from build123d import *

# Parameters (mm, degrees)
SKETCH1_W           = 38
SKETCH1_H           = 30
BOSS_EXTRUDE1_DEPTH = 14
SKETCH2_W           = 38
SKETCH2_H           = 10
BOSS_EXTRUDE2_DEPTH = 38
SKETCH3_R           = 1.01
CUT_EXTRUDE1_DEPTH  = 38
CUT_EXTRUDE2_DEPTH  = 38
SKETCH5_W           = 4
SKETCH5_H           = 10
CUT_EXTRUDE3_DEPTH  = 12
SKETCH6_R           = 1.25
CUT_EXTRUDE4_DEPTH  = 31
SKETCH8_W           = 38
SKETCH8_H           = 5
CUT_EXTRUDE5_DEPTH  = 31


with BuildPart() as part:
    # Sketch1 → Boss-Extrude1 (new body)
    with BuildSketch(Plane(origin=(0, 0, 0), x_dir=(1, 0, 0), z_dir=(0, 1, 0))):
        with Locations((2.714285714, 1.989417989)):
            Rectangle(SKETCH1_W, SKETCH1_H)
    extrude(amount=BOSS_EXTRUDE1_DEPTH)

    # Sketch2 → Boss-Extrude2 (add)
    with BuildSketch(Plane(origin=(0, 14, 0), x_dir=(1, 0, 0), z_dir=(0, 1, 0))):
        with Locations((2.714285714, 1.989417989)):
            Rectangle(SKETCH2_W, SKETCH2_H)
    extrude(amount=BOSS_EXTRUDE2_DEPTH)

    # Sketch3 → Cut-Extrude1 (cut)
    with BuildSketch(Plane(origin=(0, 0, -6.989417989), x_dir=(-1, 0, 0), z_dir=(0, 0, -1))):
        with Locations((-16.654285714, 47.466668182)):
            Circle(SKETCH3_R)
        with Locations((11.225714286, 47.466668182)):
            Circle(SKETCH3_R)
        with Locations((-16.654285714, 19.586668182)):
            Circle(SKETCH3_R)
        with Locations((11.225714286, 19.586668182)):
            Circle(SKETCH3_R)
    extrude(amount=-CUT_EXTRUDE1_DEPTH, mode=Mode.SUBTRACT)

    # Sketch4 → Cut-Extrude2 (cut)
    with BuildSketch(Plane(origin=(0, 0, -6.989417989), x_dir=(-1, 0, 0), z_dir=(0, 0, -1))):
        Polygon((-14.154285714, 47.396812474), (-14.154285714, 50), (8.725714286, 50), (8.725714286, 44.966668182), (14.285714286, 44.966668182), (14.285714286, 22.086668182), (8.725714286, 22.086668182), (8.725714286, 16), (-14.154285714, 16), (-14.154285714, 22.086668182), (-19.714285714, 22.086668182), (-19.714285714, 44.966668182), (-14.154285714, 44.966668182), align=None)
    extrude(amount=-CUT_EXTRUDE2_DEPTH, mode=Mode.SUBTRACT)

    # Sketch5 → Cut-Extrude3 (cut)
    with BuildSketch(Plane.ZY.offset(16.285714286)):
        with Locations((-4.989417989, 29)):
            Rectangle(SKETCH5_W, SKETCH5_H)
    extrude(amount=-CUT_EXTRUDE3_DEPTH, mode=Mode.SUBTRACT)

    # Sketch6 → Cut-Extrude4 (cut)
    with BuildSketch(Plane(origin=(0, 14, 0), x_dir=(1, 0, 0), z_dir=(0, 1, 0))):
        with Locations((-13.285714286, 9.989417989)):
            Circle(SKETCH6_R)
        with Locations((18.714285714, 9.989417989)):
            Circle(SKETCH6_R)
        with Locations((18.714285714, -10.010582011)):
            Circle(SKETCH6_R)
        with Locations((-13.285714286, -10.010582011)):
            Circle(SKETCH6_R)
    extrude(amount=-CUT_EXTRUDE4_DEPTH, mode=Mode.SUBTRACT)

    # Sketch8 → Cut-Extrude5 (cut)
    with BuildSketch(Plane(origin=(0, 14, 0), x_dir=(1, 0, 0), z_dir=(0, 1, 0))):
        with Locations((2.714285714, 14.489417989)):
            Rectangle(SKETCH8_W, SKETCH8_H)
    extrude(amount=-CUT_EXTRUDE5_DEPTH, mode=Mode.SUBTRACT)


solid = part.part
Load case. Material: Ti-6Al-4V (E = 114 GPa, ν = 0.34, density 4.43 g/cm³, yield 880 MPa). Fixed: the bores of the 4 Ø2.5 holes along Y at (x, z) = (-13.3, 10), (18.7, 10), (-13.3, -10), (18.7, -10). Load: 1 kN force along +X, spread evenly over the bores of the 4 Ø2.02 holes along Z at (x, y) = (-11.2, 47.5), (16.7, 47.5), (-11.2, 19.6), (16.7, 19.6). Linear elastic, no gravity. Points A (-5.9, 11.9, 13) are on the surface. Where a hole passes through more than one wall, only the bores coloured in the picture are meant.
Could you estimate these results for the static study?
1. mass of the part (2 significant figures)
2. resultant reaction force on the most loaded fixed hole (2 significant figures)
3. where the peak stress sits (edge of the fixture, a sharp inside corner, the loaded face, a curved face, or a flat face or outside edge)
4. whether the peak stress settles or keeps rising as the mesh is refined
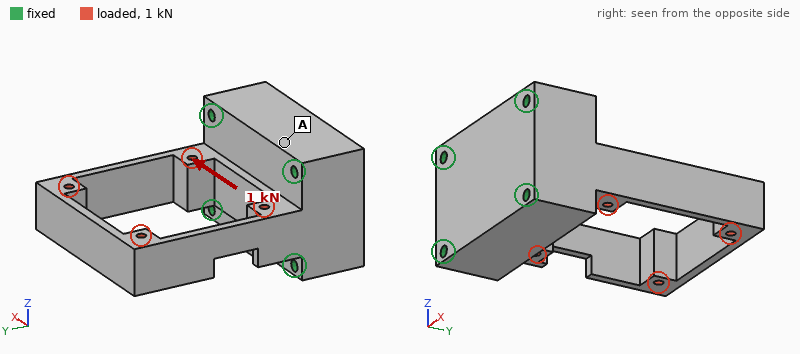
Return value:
75 g
530 N
a sharp inside corner
keeps rising
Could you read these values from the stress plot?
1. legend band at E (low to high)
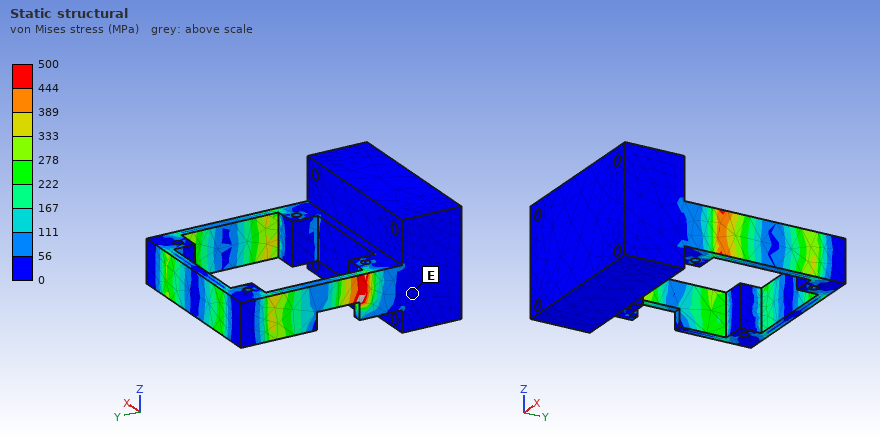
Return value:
0 to 56 MPa
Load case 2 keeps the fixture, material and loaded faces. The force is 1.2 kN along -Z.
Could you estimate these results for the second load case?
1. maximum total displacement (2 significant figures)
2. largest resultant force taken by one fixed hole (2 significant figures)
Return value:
0.51 mm
860 N
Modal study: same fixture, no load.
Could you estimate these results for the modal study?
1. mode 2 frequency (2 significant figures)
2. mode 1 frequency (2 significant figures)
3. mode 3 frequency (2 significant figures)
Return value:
2300 Hz
1600 Hz
4200 Hz
